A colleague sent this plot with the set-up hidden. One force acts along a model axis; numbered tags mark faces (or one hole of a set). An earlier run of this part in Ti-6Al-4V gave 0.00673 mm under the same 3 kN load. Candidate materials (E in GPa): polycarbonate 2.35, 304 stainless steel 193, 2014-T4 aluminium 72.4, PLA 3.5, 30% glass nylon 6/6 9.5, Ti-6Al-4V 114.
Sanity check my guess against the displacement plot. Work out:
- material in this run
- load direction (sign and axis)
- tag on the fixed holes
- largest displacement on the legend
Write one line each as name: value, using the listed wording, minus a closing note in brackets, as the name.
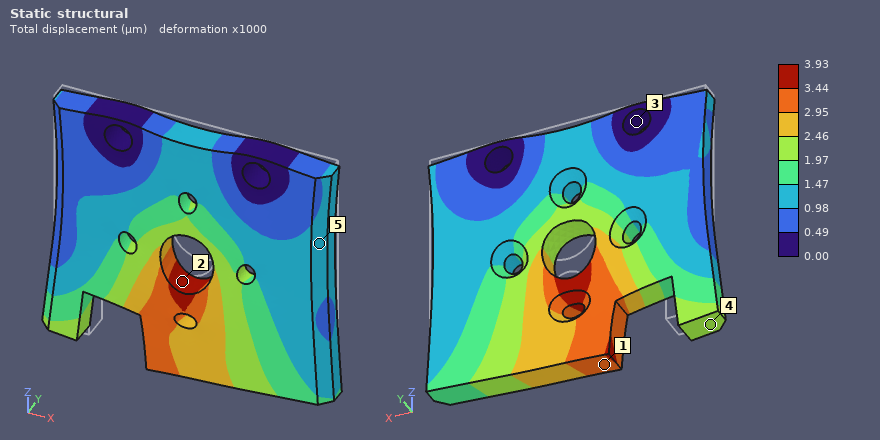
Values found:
material in this run: 304 stainless steel
load direction: -Z
tag on the fixed holes: 3
largest displacement on the legend: 3.93 µm
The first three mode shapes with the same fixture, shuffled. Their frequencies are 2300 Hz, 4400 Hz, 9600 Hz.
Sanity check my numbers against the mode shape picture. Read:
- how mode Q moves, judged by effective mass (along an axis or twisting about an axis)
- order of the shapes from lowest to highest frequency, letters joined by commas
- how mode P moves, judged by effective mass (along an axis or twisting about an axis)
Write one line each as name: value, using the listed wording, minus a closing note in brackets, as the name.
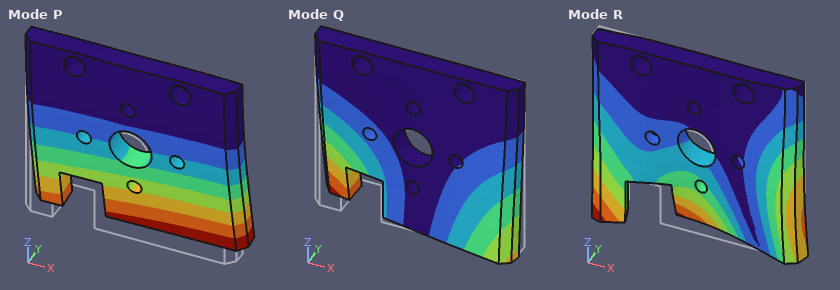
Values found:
how mode Q moves, judged by effective mass: twisting about Z
order of the shapes from lowest to highest frequency, letters joined by commas: P, Q, R
how mode P moves, judged by effective mass: along Y
